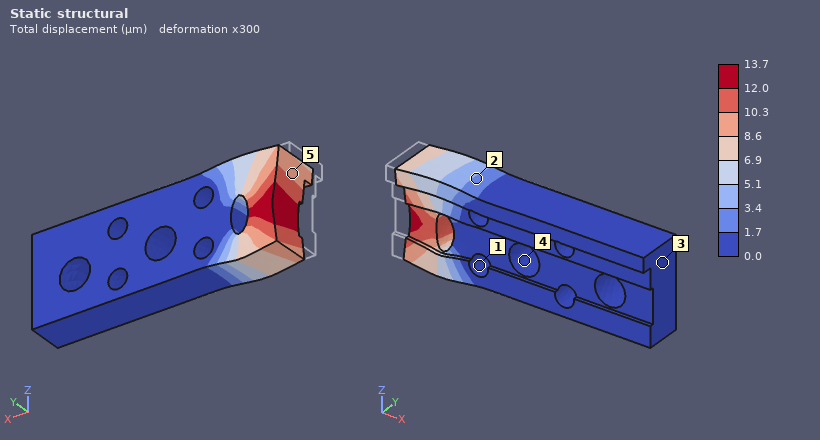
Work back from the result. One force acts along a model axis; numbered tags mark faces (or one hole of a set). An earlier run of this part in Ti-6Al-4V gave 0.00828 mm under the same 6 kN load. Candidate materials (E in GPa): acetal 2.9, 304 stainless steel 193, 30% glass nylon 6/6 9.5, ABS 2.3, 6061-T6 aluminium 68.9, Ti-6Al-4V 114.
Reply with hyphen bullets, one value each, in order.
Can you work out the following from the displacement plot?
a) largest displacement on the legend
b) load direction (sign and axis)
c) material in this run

- 13.7 µm
- +X
- 6061-T6 aluminium
